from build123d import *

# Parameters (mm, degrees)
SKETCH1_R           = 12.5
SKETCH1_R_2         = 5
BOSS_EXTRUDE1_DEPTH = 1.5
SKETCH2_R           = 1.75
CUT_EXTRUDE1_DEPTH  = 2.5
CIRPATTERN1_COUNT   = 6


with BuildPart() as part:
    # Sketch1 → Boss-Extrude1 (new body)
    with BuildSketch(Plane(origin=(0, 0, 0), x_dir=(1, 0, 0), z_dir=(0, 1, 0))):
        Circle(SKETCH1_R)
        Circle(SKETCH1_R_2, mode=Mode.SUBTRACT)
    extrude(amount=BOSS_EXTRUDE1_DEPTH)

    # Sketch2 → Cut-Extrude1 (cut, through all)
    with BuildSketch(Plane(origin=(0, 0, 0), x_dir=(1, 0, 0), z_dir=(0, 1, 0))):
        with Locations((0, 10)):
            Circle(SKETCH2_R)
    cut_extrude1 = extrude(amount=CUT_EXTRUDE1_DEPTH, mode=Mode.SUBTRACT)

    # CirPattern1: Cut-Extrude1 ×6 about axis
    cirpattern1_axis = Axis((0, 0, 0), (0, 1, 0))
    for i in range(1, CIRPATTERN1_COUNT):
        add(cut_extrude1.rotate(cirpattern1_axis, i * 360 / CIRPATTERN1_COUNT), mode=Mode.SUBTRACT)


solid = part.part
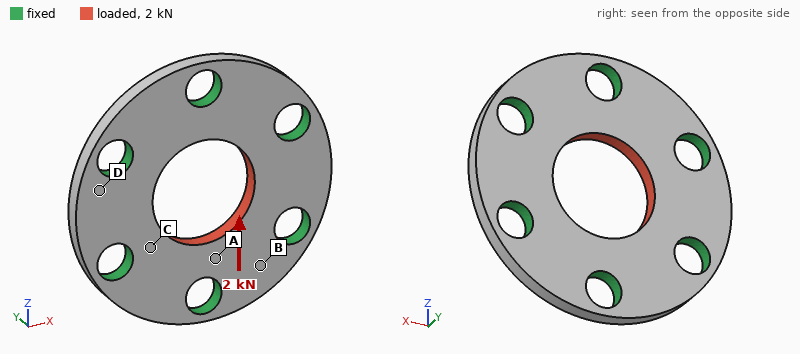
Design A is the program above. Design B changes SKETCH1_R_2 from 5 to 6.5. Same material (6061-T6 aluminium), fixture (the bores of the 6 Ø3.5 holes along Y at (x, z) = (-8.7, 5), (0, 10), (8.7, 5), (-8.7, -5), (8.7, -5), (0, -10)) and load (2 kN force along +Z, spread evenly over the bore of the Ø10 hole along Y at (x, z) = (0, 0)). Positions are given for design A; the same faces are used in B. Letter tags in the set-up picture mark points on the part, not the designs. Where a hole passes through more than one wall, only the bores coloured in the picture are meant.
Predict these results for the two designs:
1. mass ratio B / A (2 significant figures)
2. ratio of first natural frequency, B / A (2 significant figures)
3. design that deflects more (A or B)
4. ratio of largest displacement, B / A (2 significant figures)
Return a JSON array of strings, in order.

["0.85", "1.2", "A", "0.77"]
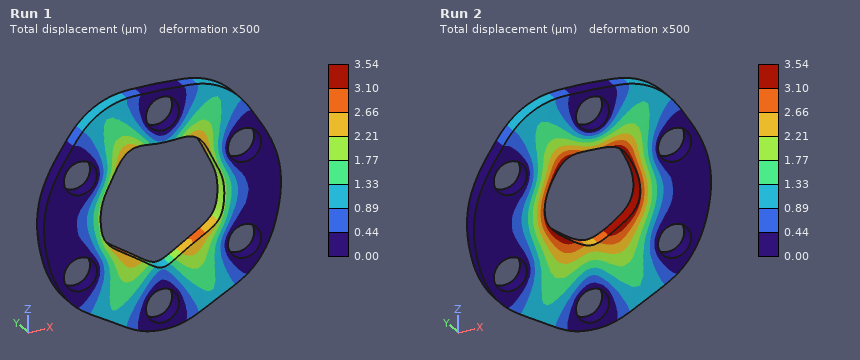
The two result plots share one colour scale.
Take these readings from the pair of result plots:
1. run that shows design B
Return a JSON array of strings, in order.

["Run 1"]
